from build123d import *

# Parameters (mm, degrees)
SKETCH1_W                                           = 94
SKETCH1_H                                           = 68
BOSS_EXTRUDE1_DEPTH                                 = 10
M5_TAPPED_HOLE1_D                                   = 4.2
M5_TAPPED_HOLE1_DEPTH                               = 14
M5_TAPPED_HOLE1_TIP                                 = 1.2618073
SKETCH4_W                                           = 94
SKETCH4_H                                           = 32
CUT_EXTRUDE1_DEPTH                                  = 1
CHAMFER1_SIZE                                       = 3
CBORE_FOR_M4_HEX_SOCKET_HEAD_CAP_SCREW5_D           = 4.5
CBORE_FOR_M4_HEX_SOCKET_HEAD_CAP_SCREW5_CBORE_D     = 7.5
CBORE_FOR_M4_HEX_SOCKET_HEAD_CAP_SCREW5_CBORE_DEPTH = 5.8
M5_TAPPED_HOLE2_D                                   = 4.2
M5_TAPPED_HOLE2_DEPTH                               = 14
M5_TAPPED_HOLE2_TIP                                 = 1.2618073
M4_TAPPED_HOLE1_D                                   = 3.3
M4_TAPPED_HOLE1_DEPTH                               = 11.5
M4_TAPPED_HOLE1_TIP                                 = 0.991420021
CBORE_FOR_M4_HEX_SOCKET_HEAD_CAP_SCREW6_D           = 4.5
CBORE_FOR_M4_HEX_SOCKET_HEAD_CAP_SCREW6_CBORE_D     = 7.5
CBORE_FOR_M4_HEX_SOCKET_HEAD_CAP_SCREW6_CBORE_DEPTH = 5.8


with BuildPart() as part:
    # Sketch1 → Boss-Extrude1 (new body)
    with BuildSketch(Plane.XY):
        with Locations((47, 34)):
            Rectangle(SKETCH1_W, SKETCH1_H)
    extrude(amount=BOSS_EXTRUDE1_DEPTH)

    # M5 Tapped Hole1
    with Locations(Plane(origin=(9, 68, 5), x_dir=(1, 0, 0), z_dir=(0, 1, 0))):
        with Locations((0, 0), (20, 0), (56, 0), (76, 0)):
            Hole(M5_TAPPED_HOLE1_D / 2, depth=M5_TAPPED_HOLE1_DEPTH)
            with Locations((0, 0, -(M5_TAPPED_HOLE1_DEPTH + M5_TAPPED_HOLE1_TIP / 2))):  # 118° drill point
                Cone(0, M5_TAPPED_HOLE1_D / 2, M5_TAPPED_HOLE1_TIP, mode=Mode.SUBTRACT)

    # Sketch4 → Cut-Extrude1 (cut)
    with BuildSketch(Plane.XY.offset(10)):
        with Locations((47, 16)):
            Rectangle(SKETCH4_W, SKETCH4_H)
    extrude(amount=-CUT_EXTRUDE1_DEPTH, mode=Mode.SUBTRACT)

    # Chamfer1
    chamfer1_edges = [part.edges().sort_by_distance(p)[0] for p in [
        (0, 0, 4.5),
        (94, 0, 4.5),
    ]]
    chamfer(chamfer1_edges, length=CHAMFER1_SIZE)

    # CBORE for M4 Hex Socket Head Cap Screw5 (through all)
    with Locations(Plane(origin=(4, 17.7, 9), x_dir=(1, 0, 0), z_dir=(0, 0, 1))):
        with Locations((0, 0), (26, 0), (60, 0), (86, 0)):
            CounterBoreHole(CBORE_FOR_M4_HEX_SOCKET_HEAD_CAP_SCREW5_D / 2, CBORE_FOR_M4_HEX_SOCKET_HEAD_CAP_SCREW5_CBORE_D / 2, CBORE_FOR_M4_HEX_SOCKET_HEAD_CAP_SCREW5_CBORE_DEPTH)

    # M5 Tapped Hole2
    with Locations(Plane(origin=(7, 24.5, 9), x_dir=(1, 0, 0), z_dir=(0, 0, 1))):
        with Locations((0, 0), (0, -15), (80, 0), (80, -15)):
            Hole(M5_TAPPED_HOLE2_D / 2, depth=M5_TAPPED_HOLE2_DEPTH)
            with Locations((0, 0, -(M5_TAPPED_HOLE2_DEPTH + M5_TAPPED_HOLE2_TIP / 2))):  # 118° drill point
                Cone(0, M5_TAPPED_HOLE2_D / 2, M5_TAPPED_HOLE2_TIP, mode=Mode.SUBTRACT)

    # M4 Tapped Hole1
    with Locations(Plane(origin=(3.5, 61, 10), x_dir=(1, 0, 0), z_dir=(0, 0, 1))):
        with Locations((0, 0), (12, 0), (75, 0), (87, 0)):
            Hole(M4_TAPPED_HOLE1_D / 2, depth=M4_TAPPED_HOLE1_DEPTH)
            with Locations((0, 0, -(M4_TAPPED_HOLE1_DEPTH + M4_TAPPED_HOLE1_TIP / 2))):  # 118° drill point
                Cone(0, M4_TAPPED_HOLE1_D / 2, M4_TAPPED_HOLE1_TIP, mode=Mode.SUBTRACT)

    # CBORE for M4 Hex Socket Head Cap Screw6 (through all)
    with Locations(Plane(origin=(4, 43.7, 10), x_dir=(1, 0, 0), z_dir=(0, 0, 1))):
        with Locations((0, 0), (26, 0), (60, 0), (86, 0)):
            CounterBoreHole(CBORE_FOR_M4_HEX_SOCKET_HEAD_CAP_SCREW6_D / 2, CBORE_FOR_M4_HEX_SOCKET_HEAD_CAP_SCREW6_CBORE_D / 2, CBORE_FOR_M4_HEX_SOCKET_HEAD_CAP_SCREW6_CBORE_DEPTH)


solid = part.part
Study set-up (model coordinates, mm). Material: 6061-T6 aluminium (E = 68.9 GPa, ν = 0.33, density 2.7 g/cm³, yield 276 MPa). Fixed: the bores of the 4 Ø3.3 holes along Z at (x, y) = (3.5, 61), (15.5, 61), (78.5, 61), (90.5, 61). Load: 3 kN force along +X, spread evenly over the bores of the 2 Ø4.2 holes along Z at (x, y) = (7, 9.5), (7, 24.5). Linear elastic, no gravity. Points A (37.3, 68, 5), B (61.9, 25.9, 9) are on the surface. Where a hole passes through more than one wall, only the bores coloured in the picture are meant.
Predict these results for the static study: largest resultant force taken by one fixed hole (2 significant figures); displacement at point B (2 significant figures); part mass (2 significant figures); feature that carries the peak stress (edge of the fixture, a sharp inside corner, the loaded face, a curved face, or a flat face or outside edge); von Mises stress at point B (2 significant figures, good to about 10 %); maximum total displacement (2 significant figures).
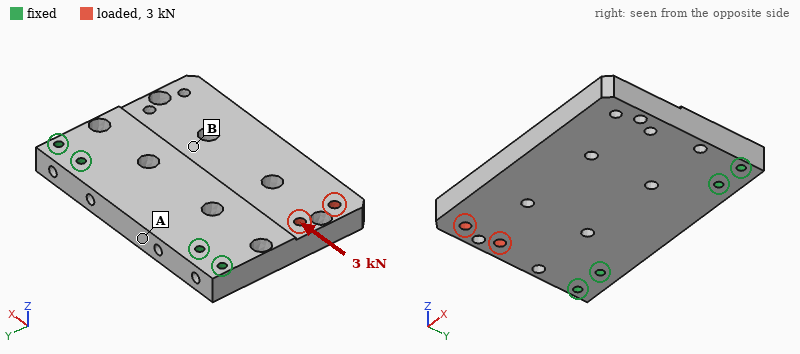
1.3 kN
6.8 µm
150 g
a curved face
7.9 MPa
17 µm
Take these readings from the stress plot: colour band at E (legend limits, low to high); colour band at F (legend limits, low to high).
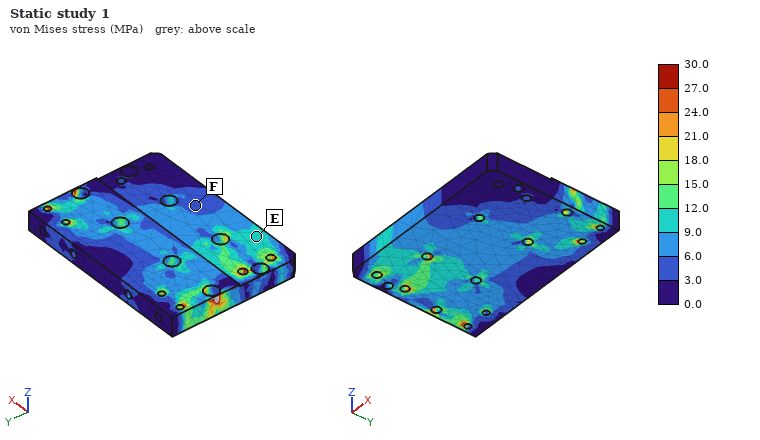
9.0 to 12.0 MPa
3.0 to 6.0 MPa
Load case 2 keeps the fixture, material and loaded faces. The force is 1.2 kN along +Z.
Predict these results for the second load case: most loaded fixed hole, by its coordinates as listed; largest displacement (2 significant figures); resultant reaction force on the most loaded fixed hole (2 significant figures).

(15.5, 61)
0.27 mm
770 N
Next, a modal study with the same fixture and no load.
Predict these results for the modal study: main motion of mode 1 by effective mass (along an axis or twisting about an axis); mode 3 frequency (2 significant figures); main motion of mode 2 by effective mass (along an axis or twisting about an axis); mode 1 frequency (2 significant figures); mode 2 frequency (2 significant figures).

along Z
7300 Hz
twisting about Y
1700 Hz
3600 Hz
